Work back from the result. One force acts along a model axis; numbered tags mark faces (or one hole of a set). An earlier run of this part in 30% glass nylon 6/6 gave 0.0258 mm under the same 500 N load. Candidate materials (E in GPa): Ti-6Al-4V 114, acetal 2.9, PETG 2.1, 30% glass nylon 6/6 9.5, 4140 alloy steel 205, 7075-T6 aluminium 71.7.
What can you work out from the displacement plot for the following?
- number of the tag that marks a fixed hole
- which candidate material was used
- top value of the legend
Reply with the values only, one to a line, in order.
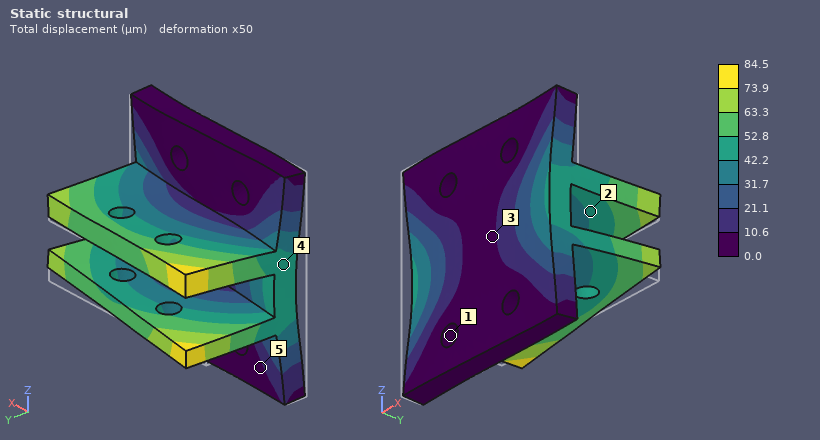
1
acetal
84.5 µm
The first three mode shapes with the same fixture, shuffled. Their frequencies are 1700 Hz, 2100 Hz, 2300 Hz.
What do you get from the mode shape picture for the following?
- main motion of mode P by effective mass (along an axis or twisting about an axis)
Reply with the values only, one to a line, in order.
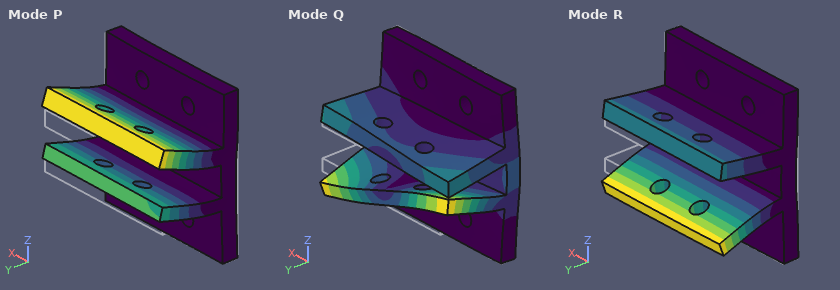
along Z
